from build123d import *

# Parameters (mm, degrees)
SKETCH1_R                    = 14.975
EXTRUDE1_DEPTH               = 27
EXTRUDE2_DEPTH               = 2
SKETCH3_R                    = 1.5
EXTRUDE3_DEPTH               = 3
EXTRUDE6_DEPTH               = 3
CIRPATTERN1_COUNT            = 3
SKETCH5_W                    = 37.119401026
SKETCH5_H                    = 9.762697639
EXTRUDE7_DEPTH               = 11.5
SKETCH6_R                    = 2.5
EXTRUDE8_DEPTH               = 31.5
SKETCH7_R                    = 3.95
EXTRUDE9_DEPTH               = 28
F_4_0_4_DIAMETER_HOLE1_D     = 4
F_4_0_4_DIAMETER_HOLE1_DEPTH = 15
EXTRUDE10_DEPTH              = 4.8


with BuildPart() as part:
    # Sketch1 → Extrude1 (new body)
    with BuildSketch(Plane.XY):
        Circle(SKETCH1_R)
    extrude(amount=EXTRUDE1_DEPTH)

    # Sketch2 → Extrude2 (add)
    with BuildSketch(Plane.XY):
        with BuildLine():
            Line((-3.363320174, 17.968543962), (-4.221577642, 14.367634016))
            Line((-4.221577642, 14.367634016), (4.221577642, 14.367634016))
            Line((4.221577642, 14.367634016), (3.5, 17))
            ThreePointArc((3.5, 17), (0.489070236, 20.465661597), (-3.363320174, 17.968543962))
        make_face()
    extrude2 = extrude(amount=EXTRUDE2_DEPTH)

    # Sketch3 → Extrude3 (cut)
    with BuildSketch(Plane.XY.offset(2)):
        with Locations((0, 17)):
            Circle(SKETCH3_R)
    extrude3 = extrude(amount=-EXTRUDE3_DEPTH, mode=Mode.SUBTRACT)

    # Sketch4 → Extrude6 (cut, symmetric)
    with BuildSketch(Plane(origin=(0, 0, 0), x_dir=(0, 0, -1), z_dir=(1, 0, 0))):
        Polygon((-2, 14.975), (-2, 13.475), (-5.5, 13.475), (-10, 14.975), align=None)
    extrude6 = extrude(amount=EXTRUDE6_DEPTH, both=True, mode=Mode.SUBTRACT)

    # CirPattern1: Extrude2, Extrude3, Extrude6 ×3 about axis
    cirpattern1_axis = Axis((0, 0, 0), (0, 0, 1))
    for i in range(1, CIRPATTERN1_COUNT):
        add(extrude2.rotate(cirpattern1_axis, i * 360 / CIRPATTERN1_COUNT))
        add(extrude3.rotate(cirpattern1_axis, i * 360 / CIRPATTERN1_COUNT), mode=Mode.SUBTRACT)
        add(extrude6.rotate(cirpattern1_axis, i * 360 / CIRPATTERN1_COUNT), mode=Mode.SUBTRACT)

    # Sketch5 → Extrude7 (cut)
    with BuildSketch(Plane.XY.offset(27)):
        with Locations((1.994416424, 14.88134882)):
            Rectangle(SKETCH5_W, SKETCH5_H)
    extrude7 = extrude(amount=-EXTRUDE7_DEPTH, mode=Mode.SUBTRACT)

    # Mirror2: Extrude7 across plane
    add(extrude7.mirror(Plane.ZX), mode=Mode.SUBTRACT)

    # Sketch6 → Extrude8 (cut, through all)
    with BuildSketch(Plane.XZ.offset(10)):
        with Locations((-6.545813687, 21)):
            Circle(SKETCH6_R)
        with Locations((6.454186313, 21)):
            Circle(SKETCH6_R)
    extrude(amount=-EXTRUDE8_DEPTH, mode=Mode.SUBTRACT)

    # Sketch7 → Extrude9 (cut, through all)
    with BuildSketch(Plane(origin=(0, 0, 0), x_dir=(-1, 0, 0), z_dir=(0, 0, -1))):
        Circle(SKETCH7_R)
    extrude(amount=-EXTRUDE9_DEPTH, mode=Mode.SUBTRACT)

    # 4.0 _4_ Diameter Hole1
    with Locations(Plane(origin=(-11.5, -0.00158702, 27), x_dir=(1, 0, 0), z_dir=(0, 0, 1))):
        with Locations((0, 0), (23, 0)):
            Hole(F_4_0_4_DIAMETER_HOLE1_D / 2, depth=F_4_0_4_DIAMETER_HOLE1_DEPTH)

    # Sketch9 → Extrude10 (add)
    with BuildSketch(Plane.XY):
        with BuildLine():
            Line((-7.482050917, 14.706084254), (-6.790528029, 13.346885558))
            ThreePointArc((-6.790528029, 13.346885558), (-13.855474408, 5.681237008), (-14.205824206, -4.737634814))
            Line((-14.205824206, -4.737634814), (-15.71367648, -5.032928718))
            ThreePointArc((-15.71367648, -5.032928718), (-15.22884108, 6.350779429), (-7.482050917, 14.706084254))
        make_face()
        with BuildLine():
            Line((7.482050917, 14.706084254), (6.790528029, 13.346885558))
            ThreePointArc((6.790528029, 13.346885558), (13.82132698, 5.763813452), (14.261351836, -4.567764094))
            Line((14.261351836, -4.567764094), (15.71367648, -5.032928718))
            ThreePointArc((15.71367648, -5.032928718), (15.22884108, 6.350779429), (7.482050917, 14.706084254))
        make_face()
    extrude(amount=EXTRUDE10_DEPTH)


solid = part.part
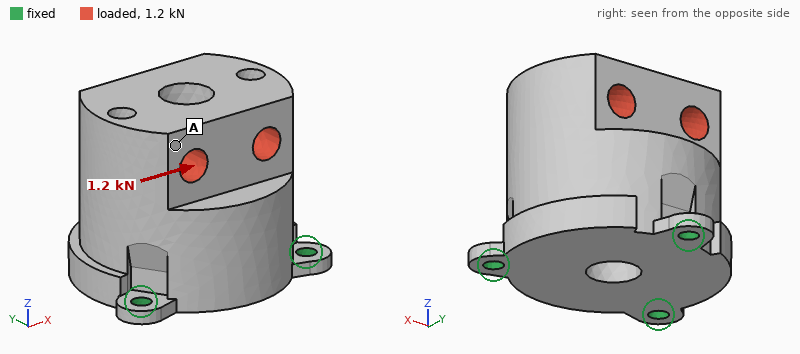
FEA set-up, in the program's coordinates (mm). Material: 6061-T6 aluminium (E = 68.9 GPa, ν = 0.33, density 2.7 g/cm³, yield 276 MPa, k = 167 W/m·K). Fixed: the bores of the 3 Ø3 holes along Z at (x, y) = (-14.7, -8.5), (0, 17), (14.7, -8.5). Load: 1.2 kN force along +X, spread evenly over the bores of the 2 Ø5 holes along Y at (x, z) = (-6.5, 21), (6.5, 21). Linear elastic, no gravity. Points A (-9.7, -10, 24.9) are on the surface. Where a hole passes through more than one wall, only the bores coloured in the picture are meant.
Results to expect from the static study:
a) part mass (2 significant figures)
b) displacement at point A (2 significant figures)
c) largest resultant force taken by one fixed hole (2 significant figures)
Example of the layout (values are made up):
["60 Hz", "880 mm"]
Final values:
["41 g", "35 µm", "1.1 kN"]
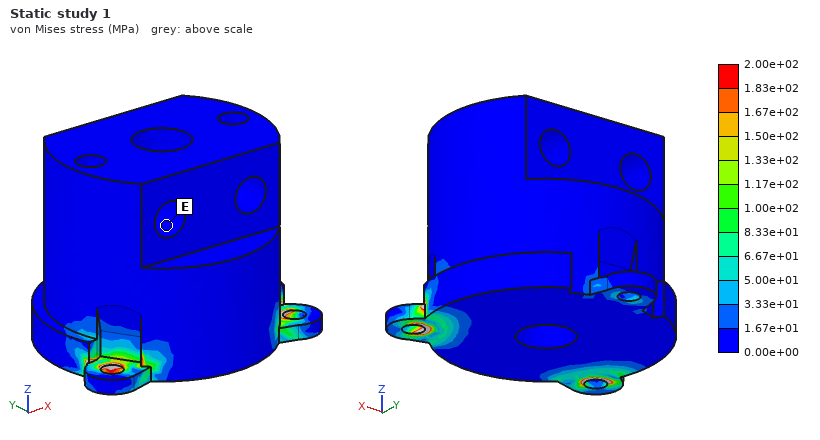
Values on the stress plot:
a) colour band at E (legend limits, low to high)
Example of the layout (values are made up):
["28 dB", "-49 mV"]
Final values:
["0.00e+00 to 1.67e+01 MPa"]
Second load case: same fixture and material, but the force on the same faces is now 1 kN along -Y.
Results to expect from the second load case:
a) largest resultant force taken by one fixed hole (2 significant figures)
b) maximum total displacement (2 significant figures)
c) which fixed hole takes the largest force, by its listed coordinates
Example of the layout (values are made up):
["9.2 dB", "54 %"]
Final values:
["1.0 kN", "36 µm", "(0, 17)"]
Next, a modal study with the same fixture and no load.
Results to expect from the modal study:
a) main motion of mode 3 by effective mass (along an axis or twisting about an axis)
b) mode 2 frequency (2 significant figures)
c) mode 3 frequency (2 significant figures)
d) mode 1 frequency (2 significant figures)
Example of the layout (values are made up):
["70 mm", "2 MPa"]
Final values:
["along Z", "6800 Hz", "10 kHz", "6600 Hz"]
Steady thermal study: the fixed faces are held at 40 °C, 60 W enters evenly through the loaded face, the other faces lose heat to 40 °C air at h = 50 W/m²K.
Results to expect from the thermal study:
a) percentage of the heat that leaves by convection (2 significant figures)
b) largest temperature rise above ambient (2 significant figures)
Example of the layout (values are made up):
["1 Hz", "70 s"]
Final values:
["13 %", "41 K"]
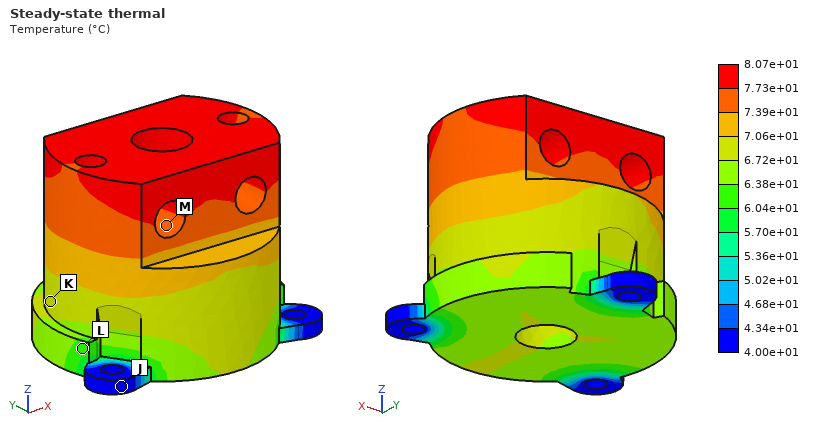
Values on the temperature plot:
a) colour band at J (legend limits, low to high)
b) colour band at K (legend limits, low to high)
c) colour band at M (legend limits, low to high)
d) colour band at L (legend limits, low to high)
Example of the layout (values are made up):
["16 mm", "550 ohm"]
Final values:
["4.00e+01 to 4.34e+01 °C", "6.72e+01 to 7.06e+01 °C", "7.39e+01 to 7.73e+01 °C", "6.04e+01 to 6.38e+01 °C"]
